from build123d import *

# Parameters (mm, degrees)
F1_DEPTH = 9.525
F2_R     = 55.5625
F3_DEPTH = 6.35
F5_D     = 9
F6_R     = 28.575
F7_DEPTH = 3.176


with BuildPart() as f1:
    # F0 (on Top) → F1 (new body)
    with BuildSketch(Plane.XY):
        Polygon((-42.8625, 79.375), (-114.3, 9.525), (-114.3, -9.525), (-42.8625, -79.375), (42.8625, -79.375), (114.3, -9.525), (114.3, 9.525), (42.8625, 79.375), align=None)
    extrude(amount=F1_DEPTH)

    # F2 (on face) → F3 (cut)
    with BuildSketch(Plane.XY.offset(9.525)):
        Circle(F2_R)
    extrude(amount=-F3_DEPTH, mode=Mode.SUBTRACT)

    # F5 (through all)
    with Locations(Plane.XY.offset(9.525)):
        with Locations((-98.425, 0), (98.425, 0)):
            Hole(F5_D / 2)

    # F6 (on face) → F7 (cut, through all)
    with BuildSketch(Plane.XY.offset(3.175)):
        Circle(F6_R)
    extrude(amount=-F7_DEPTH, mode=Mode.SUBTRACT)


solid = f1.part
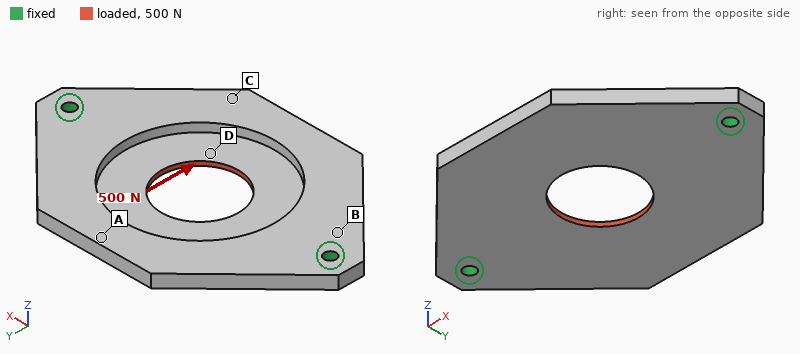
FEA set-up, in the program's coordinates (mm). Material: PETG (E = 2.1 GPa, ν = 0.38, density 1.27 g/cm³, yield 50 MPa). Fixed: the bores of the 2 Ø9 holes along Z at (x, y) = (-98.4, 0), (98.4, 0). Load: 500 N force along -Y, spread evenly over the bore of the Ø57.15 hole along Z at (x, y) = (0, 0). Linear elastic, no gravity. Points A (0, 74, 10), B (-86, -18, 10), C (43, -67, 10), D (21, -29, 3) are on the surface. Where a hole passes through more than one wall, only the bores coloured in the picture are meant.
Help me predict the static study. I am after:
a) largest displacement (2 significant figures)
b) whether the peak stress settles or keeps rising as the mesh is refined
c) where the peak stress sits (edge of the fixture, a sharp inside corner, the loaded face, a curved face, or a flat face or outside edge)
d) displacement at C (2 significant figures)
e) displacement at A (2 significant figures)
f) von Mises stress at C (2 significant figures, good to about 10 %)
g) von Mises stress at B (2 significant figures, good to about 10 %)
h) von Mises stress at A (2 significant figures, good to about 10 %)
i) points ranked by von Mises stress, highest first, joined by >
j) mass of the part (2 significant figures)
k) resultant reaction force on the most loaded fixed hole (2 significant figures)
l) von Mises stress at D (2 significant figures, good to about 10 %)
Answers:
0.27 mm
keeps rising
edge of the fixture
0.19 mm
0.24 mm
0.52 MPa
0.21 MPa
0.74 MPa
D > A > C > B
230 g
250 N
1.1 MPa
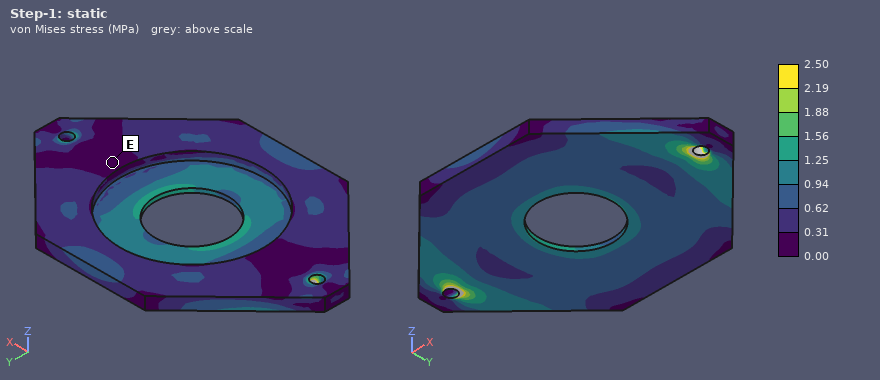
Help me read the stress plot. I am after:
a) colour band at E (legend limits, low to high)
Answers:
0.00 to 0.31 MPa
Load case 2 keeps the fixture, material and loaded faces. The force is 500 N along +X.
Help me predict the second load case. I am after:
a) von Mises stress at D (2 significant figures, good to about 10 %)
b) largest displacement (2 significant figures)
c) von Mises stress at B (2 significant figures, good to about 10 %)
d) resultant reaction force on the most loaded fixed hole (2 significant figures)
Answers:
1.1 MPa
60 µm
0.35 MPa
250 N
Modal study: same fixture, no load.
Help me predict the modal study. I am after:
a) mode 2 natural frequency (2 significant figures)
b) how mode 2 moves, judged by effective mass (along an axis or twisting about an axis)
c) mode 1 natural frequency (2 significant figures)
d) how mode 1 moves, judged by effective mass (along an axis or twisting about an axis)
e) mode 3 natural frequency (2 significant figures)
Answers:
220 Hz
along Z
180 Hz
twisting about X
490 Hz
